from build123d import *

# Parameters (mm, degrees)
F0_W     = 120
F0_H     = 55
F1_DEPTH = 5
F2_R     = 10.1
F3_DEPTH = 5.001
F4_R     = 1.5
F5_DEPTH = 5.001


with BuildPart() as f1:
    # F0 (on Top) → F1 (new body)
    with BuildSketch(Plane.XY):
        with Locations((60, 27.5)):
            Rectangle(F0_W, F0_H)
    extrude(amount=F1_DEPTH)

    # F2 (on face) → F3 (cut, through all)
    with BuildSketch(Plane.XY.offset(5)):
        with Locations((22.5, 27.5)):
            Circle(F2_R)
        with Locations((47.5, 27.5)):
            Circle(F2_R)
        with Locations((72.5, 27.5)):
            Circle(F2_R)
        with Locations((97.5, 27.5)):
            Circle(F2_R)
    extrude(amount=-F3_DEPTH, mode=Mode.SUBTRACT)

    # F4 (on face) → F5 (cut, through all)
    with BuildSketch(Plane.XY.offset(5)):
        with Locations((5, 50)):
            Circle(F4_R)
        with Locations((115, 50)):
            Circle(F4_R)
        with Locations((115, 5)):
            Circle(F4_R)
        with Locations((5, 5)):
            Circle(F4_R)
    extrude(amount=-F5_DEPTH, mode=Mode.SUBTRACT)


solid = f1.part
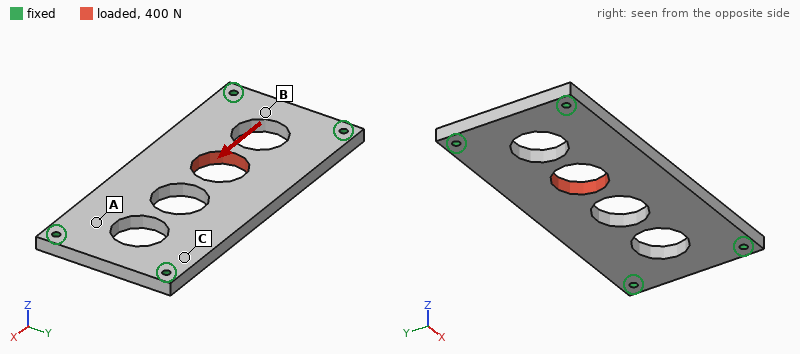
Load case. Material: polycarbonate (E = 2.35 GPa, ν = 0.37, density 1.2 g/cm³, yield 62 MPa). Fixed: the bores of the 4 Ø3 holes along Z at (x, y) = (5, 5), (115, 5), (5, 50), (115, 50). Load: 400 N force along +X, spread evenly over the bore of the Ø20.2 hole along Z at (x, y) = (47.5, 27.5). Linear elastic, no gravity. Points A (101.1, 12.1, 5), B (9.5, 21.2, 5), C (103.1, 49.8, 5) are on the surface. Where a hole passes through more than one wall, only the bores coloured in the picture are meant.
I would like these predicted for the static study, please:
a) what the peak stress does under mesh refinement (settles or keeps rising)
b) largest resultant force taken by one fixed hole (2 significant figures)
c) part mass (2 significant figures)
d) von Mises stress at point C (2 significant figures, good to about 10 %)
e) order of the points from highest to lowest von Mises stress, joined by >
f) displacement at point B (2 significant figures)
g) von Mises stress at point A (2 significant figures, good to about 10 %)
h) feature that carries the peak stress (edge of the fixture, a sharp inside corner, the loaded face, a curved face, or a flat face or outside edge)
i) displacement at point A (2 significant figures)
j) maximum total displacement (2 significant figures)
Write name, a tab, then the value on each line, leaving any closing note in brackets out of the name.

what the peak stress does under mesh refinement	keeps rising
largest resultant force taken by one fixed hole	130 N
part mass	32 g
von Mises stress at point C	1.2 MPa
order of the points from highest to lowest von Mises stress, joined by >	C > A > B
displacement at point B	9.8 µm
von Mises stress at point A	0.79 MPa
feature that carries the peak stress	edge of the fixture
displacement at point A	8.2 µm
maximum total displacement	47 µm
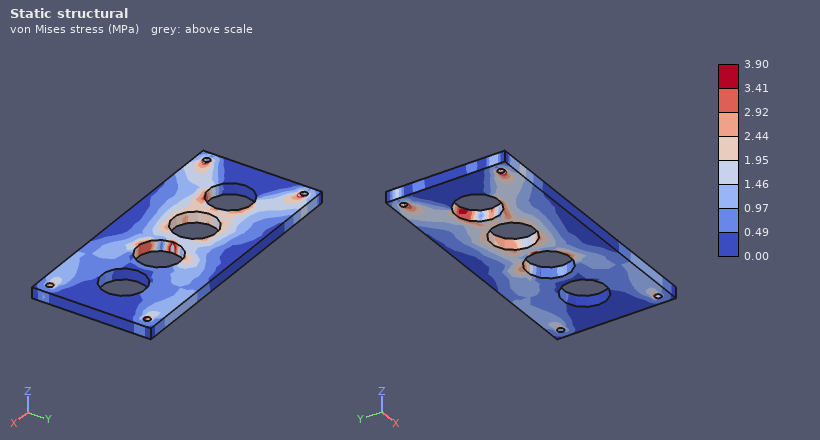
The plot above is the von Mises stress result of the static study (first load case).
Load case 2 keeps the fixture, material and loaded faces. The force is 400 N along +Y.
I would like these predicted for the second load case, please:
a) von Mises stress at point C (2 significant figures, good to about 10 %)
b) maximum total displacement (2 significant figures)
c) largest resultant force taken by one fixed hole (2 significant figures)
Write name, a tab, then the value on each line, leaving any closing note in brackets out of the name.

von Mises stress at point C	1.9 MPa
maximum total displacement	0.16 mm
largest resultant force taken by one fixed hole	180 N
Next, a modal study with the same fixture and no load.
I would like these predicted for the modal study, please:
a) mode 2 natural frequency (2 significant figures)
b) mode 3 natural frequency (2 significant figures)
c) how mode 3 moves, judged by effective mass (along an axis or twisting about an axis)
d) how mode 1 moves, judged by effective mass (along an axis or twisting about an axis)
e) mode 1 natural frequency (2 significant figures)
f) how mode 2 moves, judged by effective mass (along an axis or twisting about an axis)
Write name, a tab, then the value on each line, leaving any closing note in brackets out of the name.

mode 2 natural frequency	840 Hz
mode 3 natural frequency	1400 Hz
how mode 3 moves, judged by effective mass	twisting about Y
how mode 1 moves, judged by effective mass	along Z
mode 1 natural frequency	520 Hz
how mode 2 moves, judged by effective mass	twisting about X
